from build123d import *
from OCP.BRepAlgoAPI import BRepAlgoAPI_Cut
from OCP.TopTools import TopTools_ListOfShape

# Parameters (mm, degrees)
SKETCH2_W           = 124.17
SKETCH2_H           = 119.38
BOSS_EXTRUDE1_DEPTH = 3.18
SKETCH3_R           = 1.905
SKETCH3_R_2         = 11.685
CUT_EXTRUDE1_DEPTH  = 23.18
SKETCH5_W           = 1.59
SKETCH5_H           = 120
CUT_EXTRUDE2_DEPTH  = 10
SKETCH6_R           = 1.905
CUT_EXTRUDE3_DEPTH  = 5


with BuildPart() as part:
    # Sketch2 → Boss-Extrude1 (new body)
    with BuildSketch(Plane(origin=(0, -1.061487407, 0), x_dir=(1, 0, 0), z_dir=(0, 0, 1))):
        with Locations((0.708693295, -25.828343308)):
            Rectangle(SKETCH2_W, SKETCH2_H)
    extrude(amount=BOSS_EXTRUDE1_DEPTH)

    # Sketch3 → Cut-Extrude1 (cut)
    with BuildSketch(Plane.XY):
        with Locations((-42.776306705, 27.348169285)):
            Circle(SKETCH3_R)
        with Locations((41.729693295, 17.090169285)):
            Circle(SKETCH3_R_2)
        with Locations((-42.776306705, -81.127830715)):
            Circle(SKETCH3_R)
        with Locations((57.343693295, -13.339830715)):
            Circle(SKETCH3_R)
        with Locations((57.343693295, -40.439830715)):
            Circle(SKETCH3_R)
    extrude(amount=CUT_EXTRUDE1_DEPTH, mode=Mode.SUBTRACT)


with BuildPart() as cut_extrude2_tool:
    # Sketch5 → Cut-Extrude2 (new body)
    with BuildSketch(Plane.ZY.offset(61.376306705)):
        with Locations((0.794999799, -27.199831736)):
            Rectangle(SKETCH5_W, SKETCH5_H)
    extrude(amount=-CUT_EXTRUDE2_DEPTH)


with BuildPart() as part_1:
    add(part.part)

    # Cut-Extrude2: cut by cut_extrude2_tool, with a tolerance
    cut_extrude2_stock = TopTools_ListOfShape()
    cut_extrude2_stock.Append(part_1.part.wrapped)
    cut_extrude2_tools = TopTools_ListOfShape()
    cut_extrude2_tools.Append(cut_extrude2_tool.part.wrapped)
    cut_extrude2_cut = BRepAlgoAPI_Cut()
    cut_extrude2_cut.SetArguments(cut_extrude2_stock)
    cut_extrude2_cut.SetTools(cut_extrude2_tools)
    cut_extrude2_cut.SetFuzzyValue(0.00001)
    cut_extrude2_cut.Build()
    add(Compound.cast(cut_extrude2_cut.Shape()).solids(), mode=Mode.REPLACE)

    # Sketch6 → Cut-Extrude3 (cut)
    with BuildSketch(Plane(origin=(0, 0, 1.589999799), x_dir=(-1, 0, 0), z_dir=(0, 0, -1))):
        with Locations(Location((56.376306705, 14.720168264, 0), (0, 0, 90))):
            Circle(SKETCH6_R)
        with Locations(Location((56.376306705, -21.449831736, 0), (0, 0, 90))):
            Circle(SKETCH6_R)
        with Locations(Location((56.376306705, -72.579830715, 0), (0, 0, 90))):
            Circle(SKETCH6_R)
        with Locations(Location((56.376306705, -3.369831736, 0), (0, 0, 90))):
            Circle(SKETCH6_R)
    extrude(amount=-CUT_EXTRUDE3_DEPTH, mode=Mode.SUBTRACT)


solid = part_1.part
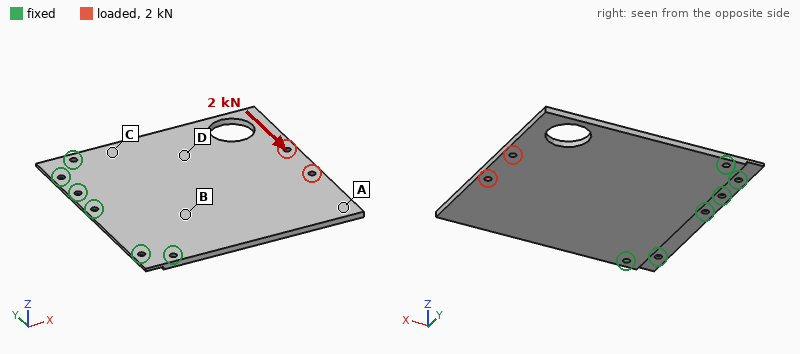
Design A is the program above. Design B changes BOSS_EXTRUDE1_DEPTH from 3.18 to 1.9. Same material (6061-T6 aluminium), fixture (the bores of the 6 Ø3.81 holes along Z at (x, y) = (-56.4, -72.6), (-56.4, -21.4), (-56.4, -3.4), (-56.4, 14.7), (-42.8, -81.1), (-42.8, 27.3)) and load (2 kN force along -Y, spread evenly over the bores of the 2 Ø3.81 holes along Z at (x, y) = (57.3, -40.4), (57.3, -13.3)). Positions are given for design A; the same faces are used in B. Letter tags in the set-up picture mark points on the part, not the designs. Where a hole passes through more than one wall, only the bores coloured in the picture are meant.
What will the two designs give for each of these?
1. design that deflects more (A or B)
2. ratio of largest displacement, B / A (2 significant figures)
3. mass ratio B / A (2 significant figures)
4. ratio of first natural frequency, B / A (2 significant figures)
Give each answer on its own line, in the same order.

B
1.9
0.58
0.58
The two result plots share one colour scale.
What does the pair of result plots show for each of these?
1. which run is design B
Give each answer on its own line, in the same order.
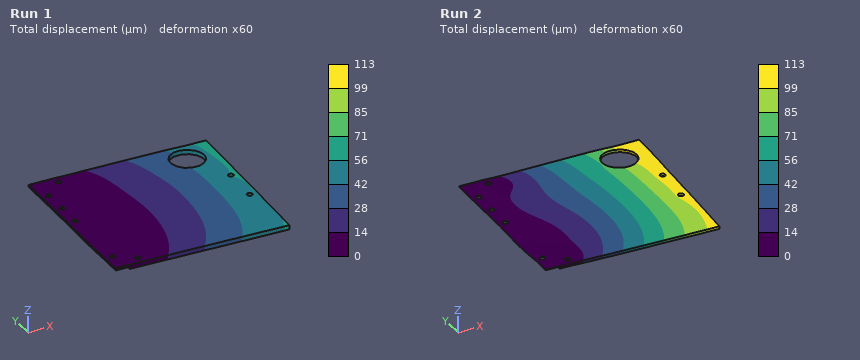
Run 2
